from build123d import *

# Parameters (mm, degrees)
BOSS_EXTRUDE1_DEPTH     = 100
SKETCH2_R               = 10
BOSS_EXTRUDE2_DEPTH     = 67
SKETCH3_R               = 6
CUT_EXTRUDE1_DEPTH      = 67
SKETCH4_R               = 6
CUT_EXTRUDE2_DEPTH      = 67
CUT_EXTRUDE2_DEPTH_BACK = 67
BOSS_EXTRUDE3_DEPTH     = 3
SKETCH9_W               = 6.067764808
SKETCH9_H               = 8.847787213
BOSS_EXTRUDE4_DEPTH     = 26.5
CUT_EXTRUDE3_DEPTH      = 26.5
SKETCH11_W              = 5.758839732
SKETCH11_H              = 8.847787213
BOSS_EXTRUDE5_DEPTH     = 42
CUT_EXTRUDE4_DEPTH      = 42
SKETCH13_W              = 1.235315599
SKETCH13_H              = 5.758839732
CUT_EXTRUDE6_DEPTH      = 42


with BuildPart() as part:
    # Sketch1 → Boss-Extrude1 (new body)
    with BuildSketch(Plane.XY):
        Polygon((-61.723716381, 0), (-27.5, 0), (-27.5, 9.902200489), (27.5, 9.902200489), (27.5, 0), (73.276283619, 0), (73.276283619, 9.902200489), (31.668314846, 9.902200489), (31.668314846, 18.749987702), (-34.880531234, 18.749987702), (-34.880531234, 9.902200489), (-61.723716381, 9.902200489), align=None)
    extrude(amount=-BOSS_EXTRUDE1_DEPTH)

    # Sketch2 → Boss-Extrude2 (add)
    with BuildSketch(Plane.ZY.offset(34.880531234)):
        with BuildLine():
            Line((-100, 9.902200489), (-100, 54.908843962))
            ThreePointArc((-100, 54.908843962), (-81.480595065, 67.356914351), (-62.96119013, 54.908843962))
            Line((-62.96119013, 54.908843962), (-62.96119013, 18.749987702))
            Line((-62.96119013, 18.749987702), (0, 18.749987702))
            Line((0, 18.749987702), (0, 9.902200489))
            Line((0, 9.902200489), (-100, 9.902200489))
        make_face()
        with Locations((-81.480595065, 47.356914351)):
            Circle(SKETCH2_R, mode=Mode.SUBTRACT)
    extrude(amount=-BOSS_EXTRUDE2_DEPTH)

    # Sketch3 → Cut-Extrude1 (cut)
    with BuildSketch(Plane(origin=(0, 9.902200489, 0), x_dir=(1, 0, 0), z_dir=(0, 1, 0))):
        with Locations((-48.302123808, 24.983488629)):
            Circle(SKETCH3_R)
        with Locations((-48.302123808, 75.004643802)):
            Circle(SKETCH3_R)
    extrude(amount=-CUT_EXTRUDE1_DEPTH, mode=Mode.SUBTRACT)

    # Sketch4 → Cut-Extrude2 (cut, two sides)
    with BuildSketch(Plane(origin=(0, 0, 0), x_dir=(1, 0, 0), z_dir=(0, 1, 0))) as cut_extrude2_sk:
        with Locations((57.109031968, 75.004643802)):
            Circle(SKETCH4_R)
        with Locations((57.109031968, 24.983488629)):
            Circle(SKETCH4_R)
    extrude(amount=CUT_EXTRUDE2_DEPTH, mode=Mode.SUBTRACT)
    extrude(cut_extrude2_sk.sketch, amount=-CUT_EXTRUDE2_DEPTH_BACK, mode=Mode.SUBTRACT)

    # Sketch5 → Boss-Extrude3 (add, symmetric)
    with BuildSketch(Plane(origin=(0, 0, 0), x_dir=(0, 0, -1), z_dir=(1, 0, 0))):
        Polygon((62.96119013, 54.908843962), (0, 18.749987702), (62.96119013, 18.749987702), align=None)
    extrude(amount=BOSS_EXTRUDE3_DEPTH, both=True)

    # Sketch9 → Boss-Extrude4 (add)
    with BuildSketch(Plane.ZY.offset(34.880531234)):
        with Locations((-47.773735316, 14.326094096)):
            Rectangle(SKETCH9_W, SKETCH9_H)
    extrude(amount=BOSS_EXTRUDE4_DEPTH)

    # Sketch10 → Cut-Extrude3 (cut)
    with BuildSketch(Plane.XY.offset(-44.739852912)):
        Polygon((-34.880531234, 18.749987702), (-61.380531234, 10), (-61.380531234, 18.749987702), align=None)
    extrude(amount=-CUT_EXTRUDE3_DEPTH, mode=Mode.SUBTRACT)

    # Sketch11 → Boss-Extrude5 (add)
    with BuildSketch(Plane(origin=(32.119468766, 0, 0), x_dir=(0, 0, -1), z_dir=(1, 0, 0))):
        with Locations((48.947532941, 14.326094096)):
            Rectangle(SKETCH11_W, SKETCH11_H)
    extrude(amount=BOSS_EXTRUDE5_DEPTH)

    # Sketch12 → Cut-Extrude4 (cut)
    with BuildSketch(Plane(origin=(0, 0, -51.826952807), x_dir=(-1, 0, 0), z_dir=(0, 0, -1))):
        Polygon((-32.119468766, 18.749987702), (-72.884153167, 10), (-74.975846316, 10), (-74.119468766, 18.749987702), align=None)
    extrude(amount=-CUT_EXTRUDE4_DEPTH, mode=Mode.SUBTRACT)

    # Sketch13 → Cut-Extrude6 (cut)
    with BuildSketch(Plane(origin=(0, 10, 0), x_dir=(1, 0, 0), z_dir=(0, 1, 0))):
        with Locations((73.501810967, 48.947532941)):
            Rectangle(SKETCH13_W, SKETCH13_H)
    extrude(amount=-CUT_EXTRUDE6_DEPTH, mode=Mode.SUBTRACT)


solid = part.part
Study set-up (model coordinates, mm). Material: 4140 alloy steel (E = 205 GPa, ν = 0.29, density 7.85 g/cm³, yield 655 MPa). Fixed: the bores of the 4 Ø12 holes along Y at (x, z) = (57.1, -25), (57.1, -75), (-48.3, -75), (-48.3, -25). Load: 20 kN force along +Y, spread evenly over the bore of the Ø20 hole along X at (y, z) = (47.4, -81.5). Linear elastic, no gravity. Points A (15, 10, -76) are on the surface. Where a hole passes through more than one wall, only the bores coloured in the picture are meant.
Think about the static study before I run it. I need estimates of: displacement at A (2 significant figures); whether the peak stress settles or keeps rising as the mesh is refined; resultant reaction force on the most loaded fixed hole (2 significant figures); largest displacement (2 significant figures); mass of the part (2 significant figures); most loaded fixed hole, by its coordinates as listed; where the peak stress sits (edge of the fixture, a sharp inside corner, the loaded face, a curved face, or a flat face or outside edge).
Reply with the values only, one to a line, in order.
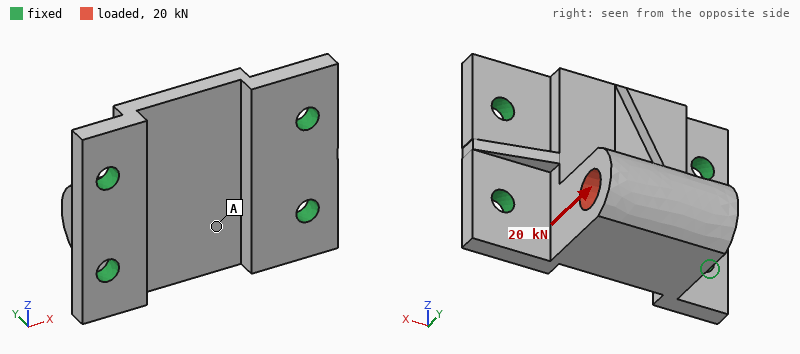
33 µm
keeps rising
16 kN
64 µm
1.8 kg
(-48.3, -75)
edge of the fixture
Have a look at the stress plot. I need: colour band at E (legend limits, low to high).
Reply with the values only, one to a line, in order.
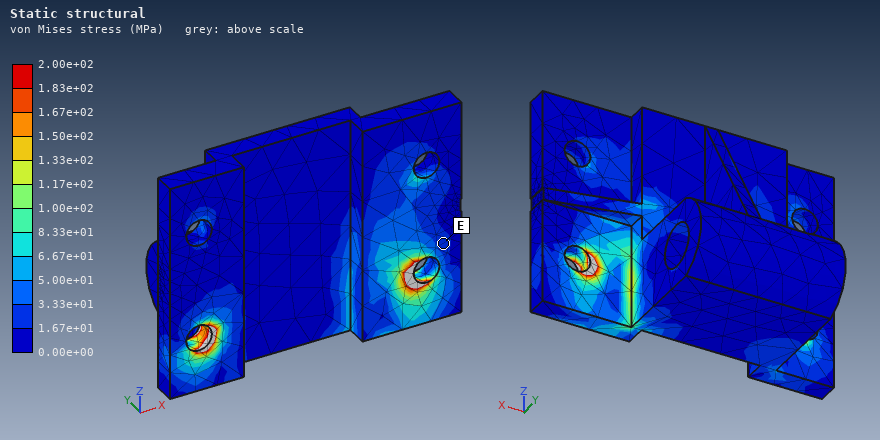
1.67e+01 to 3.33e+01 MPa
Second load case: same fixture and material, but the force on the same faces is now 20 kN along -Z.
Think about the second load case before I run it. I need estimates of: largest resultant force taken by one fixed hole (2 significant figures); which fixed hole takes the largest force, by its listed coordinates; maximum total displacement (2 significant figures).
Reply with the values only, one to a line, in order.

17 kN
(-48.3, -25)
0.11 mm
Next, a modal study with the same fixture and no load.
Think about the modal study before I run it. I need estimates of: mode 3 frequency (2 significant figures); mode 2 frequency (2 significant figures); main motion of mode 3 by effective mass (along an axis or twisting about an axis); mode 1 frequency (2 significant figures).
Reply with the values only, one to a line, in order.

5900 Hz
4000 Hz
along Y
2800 Hz
